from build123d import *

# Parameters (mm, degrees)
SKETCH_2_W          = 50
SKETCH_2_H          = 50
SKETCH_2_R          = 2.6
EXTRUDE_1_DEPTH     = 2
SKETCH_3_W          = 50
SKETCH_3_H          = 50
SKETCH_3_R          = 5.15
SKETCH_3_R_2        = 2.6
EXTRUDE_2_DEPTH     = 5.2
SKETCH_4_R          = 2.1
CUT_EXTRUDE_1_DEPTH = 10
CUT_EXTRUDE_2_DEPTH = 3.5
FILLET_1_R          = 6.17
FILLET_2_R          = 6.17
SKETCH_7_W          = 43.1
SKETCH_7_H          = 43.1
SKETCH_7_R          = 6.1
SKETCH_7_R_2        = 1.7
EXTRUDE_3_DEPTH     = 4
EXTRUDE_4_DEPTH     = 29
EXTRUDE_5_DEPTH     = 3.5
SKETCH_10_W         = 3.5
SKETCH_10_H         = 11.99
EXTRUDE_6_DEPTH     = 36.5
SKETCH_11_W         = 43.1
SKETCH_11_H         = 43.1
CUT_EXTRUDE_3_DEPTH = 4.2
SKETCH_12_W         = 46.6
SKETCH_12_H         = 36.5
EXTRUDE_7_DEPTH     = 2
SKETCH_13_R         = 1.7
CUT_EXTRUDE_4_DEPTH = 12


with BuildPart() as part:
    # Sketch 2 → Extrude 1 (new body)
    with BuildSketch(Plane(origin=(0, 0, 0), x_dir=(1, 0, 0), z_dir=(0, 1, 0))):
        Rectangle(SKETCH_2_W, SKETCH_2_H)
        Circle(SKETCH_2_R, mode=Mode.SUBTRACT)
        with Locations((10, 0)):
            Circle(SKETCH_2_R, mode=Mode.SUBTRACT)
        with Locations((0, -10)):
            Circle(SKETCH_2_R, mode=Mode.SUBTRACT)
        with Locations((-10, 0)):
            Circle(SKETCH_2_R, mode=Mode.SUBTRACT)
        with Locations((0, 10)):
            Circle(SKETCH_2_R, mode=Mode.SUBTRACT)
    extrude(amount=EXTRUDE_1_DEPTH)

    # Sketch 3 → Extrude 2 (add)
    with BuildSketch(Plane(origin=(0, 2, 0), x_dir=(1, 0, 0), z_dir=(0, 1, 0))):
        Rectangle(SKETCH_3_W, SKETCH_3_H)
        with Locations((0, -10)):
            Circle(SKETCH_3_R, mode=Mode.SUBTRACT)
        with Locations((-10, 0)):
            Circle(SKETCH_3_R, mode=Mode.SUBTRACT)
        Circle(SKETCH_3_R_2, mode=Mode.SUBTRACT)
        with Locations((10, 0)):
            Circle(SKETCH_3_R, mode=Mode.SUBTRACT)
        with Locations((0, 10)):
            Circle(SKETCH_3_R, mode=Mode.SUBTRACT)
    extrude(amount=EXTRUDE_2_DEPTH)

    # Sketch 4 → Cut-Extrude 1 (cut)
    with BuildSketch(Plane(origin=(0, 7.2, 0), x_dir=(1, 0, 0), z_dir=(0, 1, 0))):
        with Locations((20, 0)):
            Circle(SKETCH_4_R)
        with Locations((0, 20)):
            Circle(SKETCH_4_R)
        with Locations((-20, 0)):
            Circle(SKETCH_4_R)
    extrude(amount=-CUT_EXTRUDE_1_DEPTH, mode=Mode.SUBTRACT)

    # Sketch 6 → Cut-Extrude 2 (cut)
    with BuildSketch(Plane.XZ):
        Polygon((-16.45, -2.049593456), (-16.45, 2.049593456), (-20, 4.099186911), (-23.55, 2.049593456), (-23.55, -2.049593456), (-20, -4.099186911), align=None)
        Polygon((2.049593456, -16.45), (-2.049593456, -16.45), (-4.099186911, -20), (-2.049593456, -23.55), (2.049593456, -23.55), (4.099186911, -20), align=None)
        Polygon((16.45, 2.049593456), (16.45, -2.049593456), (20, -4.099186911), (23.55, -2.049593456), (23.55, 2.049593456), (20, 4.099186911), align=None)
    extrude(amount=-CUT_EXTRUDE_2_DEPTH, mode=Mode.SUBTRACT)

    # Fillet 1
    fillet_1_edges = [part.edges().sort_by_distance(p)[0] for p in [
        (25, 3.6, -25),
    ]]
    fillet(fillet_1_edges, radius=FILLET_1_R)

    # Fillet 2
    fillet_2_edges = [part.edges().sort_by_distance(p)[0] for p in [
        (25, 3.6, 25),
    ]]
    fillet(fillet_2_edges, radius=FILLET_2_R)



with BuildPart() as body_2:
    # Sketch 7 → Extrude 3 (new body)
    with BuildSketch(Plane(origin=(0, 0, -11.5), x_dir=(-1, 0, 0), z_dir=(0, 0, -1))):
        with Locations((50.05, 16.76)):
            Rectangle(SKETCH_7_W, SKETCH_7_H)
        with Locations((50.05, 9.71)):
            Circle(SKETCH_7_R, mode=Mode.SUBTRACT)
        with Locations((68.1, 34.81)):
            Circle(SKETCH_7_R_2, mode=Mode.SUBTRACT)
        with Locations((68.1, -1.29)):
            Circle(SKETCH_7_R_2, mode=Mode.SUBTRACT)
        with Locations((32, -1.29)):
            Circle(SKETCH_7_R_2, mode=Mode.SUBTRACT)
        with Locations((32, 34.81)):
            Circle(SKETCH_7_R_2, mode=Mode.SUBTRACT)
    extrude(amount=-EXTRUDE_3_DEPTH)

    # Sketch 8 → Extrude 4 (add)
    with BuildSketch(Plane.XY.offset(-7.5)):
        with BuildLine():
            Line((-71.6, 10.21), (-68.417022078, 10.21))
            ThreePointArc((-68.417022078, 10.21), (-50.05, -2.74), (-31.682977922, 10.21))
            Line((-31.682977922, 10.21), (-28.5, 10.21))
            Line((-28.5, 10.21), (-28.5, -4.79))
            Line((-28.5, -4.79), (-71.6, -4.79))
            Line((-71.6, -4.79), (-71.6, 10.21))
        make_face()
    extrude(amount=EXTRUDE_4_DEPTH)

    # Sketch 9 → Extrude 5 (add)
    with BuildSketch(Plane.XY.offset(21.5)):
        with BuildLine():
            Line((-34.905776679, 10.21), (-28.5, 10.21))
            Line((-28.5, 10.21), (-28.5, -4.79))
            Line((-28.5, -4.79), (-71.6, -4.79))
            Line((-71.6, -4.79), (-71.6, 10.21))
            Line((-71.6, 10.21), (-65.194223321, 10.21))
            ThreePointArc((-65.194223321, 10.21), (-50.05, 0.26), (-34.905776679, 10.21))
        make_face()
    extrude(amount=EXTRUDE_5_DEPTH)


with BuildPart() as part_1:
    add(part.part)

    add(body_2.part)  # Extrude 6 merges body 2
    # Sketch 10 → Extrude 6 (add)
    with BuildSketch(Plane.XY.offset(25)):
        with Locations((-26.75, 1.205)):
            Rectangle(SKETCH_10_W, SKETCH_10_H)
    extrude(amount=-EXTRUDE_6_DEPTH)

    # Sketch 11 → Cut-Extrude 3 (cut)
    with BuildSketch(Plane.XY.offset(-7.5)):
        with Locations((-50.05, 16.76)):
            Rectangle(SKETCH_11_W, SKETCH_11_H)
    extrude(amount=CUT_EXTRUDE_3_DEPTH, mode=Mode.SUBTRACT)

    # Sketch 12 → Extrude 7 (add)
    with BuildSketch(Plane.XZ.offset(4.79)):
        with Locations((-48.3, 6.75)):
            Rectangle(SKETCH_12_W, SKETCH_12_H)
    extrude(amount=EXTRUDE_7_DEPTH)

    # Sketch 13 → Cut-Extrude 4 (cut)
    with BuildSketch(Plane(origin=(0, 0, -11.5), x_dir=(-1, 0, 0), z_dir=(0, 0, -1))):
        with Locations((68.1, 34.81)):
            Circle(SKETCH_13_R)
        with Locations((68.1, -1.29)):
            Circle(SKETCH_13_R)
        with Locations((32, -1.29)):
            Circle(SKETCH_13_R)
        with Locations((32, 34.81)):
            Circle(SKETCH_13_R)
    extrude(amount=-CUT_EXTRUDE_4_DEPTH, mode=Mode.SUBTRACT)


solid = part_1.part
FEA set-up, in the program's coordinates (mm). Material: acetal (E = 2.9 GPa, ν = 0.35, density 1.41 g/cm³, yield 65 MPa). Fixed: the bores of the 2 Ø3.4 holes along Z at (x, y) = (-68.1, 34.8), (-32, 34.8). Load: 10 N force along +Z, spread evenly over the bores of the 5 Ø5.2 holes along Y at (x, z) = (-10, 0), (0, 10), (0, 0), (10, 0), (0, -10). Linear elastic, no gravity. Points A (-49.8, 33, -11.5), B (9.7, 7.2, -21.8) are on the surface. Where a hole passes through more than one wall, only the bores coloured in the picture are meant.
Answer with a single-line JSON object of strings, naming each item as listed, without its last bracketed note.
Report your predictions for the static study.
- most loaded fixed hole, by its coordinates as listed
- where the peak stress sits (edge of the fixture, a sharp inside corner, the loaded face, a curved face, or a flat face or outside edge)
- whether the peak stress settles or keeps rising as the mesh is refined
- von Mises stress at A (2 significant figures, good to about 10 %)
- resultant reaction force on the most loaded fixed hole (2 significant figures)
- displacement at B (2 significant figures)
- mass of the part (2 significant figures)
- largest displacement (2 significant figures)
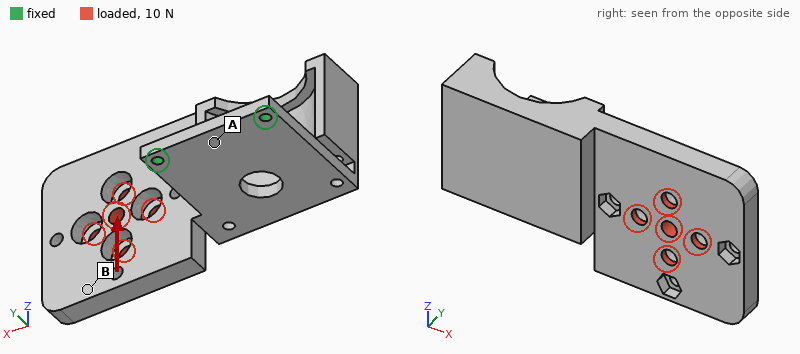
{"most loaded fixed hole, by its coordinates as listed": "(-32, 34.8)", "where the peak stress sits": "edge of the fixture", "whether the peak stress settles or keeps rising as the mesh is refined": "keeps rising", "von Mises stress at A": "1.2 MPa", "resultant reaction force on the most loaded fixed hole": "19 N", "displacement at B": "0.94 mm", "mass of the part": "51 g", "largest displacement": "1.4 mm"}
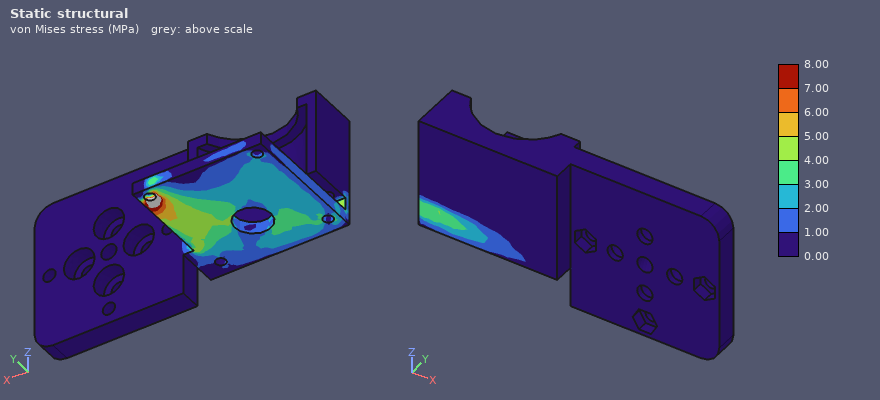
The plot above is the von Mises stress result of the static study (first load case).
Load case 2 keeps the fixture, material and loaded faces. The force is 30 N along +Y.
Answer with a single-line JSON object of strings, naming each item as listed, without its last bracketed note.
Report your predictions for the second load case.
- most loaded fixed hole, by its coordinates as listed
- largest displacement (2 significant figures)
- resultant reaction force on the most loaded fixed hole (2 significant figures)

{"most loaded fixed hole, by its coordinates as listed": "(-32, 34.8)", "largest displacement": "1.3 mm", "resultant reaction force on the most loaded fixed hole": "57 N"}
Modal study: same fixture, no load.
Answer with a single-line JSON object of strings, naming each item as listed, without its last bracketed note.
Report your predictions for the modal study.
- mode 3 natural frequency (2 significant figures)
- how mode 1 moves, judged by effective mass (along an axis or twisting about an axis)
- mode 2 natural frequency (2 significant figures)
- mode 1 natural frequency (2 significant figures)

{"mode 3 natural frequency": "310 Hz", "how mode 1 moves, judged by effective mass": "along Z", "mode 2 natural frequency": "150 Hz", "mode 1 natural frequency": "90 Hz"}
